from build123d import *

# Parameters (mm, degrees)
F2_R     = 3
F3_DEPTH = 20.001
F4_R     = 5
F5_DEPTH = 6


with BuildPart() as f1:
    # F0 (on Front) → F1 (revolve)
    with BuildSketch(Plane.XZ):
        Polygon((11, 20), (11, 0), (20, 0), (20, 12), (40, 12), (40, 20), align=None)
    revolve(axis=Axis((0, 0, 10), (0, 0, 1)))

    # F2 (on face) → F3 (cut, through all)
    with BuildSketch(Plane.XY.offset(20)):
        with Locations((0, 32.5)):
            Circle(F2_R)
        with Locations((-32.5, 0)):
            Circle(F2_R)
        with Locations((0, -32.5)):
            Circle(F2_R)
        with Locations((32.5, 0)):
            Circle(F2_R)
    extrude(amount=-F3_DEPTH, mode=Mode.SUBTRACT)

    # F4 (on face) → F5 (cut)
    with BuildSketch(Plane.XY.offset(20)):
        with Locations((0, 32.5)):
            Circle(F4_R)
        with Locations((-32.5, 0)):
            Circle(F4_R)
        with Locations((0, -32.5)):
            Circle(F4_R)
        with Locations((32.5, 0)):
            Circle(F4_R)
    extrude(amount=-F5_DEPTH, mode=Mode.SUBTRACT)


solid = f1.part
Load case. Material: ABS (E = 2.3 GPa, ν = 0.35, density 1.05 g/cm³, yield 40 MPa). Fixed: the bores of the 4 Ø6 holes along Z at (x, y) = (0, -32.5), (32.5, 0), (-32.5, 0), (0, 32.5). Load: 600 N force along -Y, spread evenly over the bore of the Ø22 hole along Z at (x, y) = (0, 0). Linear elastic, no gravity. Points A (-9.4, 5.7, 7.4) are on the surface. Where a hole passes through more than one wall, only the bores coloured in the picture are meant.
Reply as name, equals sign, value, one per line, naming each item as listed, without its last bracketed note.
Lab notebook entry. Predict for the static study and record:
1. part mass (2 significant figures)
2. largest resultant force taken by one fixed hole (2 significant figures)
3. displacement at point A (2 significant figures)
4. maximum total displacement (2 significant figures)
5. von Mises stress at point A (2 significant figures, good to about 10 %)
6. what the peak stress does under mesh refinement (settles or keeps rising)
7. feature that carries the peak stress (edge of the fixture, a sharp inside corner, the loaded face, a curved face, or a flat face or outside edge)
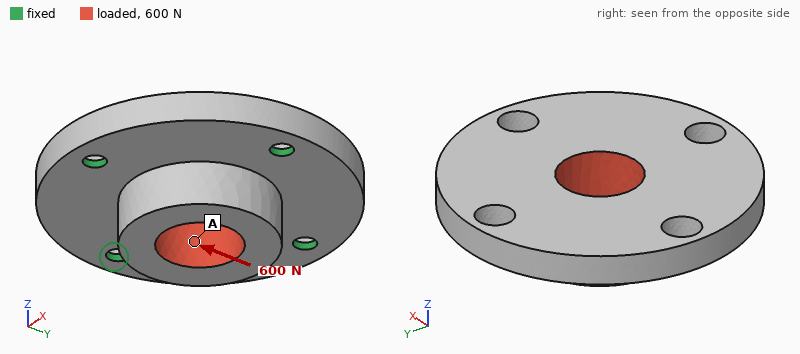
part mass = 48 g
largest resultant force taken by one fixed hole = 160 N
displacement at point A = 29 µm
maximum total displacement = 41 µm
von Mises stress at point A = 0.91 MPa
what the peak stress does under mesh refinement = keeps rising
feature that carries the peak stress = edge of the fixture
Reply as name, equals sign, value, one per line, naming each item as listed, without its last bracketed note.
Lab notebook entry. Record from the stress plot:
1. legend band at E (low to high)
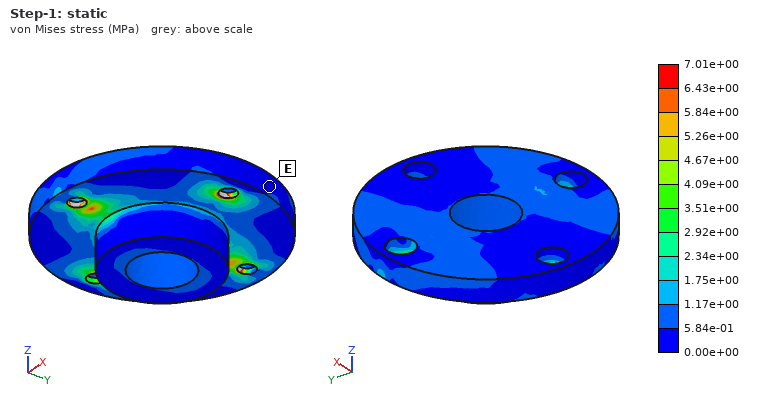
legend band at E = 0.00e+00 to 5.84e-01 MPa
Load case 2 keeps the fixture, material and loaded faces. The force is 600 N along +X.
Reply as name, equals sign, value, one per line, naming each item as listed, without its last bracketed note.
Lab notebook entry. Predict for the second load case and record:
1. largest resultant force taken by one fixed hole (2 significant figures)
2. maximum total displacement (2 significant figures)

largest resultant force taken by one fixed hole = 160 N
maximum total displacement = 41 µm
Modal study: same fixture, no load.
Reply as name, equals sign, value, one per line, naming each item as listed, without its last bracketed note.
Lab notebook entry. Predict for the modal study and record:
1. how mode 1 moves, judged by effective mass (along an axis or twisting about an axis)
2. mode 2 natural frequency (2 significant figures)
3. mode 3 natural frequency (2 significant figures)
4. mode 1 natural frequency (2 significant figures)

how mode 1 moves, judged by effective mass = along Z
mode 2 natural frequency = 2900 Hz
mode 3 natural frequency = 2900 Hz
mode 1 natural frequency = 2600 Hz
